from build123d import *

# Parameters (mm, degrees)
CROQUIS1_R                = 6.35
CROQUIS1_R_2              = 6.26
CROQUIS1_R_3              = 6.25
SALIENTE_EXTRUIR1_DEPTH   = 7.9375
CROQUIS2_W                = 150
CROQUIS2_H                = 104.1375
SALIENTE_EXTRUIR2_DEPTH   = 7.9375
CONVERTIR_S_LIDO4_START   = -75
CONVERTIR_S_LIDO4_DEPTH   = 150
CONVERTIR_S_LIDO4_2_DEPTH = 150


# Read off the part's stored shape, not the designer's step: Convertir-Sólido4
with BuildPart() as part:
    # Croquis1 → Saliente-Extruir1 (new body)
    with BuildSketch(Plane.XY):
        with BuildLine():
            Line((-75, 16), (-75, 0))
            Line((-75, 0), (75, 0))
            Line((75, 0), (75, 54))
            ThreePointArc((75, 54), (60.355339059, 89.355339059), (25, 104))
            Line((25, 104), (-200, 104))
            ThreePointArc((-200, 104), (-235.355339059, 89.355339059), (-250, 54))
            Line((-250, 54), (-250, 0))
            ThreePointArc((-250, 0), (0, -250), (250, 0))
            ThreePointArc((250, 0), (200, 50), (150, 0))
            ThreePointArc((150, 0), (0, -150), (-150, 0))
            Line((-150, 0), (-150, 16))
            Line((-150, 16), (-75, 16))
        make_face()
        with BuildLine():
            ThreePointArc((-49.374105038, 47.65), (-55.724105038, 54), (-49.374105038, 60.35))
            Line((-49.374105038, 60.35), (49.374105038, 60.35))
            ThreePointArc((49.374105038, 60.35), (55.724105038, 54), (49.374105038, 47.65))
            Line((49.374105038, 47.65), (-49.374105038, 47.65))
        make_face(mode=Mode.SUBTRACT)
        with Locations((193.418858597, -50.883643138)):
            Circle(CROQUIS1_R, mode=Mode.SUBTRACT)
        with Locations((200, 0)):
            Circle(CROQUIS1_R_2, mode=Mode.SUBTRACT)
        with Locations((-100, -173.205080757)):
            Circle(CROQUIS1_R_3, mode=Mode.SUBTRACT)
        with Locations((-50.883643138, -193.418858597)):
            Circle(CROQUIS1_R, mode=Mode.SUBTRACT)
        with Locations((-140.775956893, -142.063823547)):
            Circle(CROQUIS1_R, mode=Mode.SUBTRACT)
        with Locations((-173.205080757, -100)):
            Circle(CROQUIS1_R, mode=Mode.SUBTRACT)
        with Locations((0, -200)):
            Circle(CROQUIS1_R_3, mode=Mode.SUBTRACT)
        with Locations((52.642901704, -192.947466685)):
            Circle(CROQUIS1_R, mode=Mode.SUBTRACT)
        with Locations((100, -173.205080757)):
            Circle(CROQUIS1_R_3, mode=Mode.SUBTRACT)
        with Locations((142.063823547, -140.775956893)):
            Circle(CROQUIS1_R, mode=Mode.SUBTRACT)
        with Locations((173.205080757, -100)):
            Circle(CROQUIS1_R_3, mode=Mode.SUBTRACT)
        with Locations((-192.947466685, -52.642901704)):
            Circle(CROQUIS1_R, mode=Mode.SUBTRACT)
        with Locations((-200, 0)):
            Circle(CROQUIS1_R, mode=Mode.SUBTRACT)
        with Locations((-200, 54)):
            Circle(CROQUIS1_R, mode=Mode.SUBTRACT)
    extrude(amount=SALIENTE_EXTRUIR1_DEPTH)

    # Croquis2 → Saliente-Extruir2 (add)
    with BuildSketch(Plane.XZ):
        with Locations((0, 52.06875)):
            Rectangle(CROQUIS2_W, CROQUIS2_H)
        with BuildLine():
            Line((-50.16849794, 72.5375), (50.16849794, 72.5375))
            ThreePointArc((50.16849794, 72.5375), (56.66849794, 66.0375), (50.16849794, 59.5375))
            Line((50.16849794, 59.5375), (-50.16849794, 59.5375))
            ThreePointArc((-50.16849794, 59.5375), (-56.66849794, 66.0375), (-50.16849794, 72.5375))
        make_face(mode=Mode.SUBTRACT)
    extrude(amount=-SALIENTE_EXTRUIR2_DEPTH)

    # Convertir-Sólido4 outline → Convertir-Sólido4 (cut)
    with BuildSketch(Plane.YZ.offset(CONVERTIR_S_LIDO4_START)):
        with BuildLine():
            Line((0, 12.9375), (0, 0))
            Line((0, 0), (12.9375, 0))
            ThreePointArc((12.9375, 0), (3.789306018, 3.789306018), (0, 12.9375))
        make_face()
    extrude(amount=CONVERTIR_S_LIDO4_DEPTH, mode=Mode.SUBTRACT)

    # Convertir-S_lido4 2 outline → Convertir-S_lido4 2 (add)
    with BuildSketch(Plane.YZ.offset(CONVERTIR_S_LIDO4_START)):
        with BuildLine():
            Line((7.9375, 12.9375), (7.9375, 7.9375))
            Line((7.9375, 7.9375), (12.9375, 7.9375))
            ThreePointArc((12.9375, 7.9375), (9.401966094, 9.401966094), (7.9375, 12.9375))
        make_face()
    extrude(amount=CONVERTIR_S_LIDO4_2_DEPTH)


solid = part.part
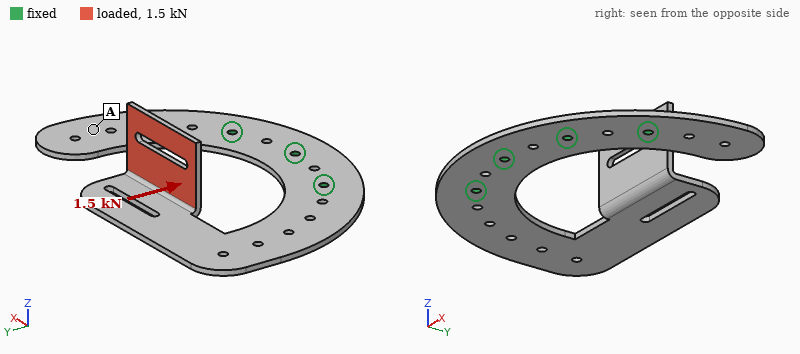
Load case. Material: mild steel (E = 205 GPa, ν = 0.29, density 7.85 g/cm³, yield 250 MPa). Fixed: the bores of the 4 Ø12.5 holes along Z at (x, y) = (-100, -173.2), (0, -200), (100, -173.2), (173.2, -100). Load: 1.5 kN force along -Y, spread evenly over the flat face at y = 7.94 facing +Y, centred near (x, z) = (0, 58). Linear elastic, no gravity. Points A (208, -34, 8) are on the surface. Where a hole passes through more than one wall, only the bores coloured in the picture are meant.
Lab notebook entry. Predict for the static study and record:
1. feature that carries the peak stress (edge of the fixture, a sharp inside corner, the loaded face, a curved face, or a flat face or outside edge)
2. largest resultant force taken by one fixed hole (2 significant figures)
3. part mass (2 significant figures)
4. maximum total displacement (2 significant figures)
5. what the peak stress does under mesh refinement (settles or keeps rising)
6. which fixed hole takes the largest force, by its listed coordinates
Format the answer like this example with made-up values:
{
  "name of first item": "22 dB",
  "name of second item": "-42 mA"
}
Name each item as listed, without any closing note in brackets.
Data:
{
  "feature that carries the peak stress": "a sharp inside corner",
  "largest resultant force taken by one fixed hole": "1.1 kN",
  "part mass": "6.7 kg",
  "maximum total displacement": "4.3 mm",
  "what the peak stress does under mesh refinement": "keeps rising",
  "which fixed hole takes the largest force, by its listed coordinates": "(0, -200)"
}
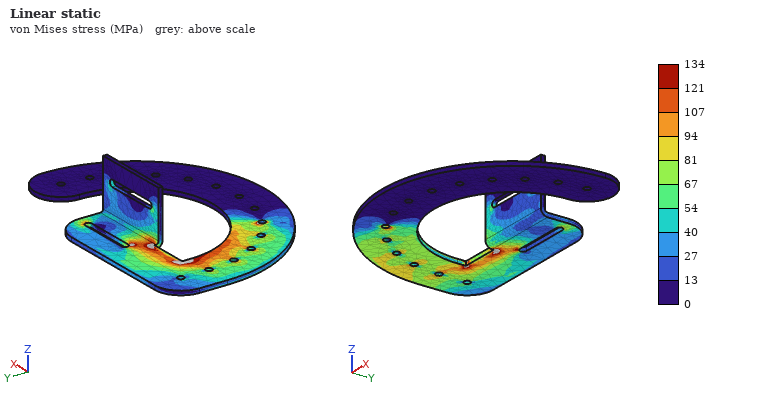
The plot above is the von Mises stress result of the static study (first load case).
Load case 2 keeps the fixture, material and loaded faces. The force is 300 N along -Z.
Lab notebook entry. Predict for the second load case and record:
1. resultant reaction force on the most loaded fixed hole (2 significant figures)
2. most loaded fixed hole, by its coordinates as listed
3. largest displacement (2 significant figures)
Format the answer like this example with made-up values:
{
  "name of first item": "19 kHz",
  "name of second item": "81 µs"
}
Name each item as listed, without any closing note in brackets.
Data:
{
  "resultant reaction force on the most loaded fixed hole": "290 N",
  "most loaded fixed hole, by its coordinates as listed": "(-100, -173.2)",
  "largest displacement": "4.5 mm"
}
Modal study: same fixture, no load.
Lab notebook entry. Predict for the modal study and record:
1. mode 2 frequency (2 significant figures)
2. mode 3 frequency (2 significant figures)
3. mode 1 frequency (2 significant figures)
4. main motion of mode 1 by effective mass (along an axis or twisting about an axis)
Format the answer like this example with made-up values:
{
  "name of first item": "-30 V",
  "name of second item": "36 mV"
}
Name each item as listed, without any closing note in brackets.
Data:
{
  "mode 2 frequency": "61 Hz",
  "mode 3 frequency": "160 Hz",
  "mode 1 frequency": "35 Hz",
  "main motion of mode 1 by effective mass": "along Z"
}
